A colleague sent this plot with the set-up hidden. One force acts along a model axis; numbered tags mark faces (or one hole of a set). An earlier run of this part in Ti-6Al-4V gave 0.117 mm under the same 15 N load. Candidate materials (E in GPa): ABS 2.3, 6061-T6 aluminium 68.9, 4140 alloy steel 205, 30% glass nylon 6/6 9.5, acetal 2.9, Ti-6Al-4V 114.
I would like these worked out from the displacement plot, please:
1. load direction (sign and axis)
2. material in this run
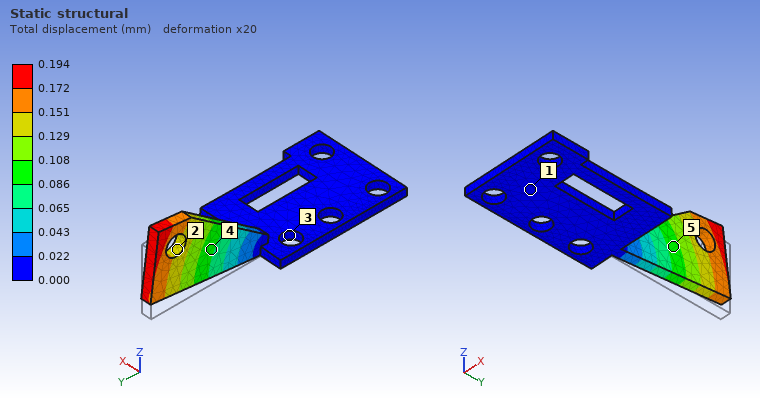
+Z
6061-T6 aluminium
